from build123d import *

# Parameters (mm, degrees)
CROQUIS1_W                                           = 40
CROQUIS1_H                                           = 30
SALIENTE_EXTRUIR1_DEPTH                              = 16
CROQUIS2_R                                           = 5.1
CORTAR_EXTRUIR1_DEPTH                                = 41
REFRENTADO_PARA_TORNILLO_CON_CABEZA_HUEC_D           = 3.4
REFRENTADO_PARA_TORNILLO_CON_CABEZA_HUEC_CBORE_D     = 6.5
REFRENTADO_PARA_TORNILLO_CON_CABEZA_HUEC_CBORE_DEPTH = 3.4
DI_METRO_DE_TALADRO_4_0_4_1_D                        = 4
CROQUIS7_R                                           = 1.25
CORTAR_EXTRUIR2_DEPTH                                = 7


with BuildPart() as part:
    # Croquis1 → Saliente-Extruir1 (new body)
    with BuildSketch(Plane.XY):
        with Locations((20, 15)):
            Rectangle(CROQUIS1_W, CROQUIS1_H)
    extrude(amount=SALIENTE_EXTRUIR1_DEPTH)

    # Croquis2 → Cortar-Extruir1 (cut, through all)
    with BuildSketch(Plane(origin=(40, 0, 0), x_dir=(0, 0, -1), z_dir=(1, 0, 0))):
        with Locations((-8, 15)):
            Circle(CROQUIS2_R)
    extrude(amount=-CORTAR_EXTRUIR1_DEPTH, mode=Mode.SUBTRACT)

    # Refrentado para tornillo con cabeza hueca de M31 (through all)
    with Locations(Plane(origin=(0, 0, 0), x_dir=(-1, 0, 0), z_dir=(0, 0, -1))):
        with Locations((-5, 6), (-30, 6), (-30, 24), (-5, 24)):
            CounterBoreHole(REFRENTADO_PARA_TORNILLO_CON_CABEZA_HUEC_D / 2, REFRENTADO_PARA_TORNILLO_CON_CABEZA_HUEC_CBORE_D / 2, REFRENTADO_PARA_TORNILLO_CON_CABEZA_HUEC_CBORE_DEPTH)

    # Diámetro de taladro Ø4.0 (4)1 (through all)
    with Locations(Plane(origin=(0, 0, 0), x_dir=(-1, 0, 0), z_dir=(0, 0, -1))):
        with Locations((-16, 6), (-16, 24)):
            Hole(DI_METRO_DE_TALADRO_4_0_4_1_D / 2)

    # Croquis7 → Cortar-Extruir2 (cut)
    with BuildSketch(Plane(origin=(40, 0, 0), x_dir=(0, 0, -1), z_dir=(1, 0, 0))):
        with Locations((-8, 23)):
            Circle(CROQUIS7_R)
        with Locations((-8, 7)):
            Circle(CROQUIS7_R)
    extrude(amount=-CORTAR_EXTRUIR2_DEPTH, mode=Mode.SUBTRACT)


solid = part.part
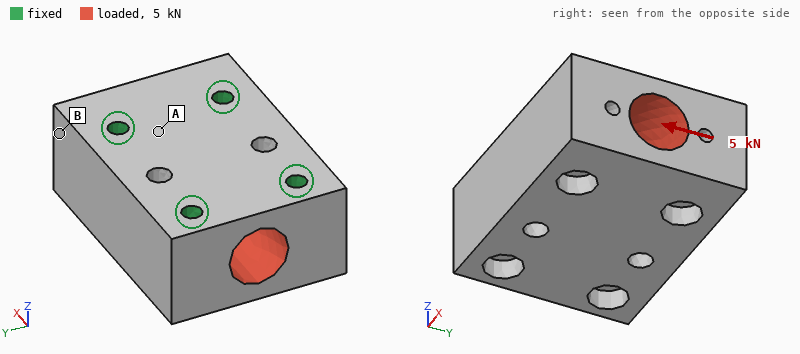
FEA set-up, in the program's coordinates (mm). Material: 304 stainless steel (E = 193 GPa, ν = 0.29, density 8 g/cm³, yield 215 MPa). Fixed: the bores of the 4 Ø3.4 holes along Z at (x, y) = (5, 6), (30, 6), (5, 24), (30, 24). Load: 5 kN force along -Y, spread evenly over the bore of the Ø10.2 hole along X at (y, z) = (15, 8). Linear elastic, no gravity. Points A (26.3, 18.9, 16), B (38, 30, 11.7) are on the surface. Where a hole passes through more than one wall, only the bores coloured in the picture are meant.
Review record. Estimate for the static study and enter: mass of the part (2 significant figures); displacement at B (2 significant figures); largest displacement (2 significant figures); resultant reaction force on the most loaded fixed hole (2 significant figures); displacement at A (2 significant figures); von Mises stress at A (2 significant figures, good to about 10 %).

120 g
0.32 µm
0.76 µm
1.4 kN
0.25 µm
6.0 MPa
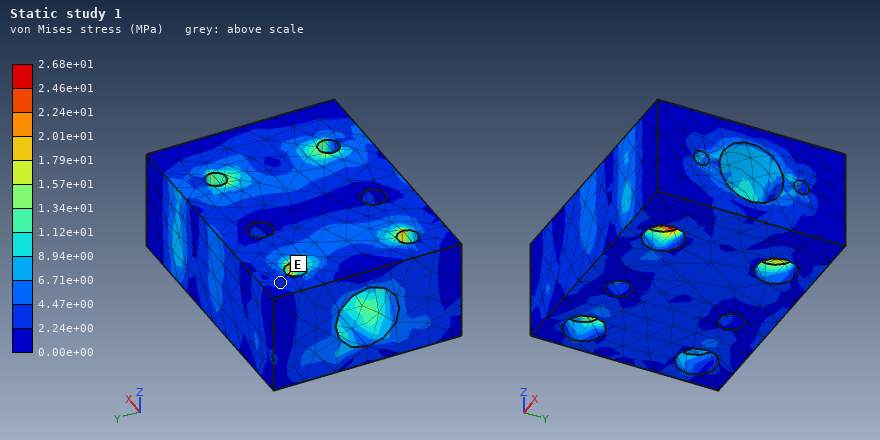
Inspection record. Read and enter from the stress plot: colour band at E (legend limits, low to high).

2.24e+00 to 4.47e+00 MPa
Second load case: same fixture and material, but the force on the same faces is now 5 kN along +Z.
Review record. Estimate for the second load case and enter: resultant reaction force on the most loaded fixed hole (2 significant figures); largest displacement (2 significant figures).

1.4 kN
1.3 µm
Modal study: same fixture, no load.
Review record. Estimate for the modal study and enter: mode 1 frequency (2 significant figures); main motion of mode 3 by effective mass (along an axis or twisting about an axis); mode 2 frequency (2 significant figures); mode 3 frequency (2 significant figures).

44 kHz
along Z
46 kHz
48 kHz
